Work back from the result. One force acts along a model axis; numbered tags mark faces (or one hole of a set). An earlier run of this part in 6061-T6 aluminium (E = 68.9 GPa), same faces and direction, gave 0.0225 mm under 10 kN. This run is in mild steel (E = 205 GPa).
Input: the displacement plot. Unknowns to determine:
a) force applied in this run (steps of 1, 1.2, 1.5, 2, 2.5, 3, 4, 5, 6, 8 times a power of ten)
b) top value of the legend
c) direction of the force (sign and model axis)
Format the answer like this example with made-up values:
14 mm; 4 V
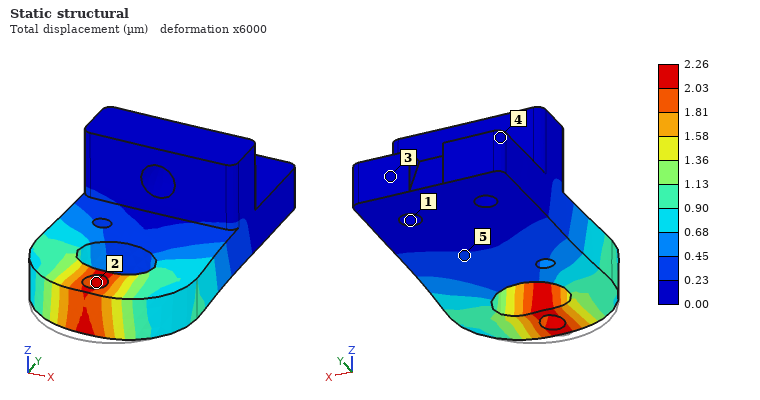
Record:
3 kN; 2.26 µm; +Y
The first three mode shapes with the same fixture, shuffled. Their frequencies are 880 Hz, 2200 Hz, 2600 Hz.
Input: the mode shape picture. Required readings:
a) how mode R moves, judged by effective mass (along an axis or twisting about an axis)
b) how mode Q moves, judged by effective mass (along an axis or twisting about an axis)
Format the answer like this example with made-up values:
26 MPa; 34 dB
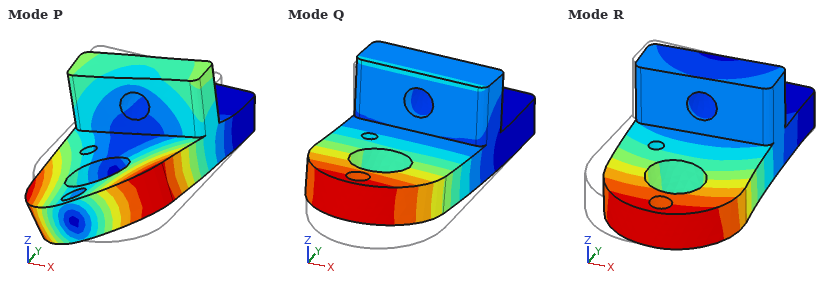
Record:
along X; along Z
